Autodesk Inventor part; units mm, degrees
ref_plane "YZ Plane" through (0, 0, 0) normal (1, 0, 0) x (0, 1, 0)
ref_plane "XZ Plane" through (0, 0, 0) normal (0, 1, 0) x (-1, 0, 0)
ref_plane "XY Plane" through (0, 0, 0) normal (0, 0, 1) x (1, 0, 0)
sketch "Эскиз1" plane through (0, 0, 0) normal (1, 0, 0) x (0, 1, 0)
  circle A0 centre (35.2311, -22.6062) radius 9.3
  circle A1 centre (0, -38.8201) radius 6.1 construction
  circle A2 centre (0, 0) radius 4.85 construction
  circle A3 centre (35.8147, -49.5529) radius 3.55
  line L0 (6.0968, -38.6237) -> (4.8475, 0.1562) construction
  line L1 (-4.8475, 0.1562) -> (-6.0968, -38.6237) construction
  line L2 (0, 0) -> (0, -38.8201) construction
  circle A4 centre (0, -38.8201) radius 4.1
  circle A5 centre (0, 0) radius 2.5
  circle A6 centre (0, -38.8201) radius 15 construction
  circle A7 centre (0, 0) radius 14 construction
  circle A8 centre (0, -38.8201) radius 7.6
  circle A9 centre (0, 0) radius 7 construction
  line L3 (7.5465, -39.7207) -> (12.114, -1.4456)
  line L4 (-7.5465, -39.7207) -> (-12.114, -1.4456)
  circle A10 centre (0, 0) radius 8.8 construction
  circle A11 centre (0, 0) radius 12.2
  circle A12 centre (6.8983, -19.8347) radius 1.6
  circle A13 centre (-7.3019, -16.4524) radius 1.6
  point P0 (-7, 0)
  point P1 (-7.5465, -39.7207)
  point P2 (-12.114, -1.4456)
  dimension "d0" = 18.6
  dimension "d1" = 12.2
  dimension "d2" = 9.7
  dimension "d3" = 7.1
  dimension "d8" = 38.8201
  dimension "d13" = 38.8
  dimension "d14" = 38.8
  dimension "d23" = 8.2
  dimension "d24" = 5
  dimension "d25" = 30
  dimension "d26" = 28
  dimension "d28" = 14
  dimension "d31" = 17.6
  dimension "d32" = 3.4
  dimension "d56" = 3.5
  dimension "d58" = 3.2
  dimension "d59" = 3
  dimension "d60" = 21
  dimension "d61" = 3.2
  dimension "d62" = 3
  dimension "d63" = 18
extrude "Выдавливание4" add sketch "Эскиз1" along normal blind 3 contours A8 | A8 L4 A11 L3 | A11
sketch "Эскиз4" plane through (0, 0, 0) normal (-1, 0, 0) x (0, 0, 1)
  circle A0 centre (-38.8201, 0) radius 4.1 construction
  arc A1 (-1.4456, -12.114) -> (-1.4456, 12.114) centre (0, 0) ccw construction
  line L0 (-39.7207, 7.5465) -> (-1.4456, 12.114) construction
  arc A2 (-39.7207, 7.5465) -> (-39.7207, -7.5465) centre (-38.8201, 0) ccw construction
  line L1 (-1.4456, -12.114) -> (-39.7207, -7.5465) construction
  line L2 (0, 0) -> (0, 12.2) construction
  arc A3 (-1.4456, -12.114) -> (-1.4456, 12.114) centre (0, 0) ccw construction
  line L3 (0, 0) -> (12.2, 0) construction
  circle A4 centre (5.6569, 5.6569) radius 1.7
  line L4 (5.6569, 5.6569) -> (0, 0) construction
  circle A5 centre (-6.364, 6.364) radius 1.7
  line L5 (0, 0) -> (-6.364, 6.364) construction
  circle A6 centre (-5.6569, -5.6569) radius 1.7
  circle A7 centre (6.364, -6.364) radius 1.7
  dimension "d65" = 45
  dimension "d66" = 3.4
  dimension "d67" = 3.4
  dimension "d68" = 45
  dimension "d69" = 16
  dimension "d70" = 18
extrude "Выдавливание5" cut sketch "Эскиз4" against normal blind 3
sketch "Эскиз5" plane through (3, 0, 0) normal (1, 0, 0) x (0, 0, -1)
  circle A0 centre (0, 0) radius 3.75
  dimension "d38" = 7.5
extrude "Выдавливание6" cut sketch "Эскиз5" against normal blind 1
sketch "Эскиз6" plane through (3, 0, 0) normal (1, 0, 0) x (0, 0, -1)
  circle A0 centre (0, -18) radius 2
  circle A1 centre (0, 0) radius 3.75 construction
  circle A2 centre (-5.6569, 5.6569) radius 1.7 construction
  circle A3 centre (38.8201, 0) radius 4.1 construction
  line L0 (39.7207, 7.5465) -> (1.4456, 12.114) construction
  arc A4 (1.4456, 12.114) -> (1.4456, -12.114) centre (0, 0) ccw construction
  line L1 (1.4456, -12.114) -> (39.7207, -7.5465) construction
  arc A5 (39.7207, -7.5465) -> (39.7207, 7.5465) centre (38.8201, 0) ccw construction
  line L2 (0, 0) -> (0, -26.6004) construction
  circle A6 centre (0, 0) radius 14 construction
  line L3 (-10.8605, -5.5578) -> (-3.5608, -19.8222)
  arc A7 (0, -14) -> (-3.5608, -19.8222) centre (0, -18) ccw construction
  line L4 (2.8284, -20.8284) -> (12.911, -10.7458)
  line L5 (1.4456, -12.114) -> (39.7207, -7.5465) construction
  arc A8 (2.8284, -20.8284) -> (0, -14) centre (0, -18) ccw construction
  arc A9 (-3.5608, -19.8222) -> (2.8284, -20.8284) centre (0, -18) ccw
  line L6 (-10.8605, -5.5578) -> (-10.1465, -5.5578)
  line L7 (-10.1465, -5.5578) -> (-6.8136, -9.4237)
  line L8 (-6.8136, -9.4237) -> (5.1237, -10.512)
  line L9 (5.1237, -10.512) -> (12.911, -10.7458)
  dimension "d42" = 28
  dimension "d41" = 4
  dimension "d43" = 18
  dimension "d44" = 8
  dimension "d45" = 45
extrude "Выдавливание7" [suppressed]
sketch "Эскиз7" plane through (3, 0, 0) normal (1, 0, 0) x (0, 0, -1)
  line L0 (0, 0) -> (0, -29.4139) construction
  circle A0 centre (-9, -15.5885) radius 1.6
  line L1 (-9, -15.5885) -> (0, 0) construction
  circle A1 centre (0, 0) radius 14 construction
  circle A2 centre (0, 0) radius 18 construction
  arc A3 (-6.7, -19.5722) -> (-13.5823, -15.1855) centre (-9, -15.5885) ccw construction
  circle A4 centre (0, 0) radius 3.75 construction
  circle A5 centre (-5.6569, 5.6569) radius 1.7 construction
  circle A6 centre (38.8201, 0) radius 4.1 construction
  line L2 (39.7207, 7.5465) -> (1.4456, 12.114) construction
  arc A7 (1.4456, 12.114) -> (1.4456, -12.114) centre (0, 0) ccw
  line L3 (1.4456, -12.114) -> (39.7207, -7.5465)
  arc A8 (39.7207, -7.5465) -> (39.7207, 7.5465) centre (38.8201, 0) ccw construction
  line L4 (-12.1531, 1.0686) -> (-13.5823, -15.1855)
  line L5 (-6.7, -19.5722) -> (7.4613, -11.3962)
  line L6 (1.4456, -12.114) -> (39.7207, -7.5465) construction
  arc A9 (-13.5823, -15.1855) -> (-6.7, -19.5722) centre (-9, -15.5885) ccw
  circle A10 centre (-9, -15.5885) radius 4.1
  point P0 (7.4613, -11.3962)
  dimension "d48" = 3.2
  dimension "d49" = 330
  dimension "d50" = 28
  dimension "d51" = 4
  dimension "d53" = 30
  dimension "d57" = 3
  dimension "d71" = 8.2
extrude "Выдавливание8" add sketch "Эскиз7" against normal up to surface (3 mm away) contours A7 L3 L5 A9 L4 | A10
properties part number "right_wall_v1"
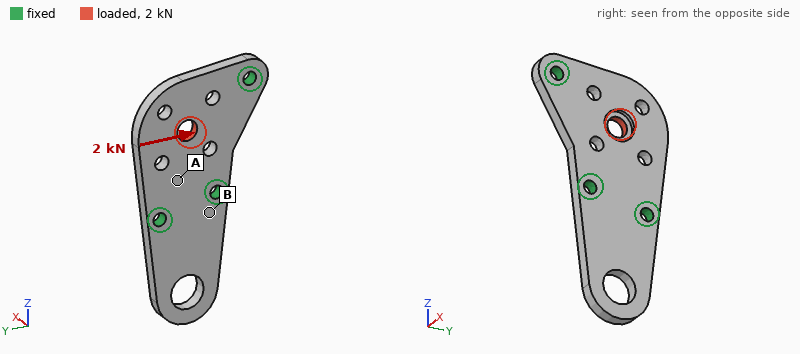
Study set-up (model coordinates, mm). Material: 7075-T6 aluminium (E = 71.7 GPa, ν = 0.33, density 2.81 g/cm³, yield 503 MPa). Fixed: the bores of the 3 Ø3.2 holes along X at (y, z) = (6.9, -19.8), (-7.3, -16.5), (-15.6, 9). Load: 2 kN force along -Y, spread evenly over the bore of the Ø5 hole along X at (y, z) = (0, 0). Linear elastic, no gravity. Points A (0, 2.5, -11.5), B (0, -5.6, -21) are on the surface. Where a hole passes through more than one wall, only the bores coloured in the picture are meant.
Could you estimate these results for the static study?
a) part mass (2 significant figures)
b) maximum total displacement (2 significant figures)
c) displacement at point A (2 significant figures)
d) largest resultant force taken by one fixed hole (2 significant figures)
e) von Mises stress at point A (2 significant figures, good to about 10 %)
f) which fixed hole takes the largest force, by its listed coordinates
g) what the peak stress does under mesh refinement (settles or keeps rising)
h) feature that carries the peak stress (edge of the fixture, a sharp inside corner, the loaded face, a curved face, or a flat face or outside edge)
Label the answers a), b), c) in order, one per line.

a) 9.2 g
b) 35 µm
c) 5.6 µm
d) 1.3 kN
e) 32 MPa
f) (-15.6, 9)
g) keeps rising
h) edge of the fixture
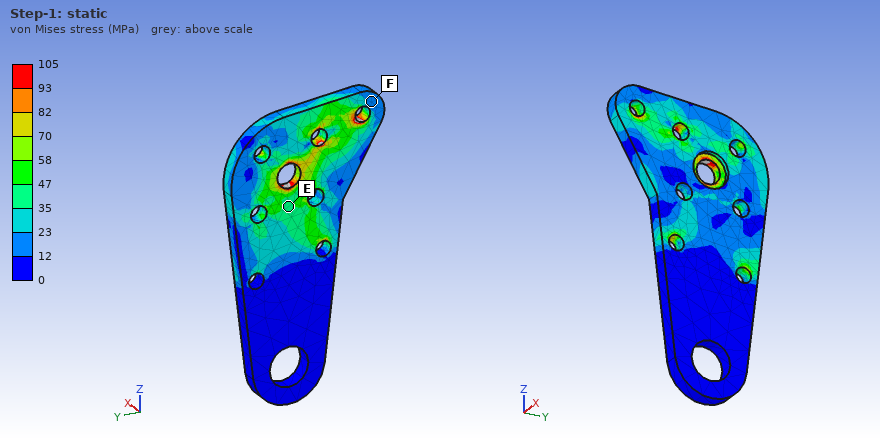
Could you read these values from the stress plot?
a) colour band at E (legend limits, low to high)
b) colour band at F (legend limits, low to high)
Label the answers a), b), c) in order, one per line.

a) 35 to 47 MPa
b) 12 to 23 MPa
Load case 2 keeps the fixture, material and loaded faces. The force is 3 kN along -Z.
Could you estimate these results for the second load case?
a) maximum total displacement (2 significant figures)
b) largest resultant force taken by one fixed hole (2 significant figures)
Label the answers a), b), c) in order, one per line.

a) 38 µm
b) 1.3 kN
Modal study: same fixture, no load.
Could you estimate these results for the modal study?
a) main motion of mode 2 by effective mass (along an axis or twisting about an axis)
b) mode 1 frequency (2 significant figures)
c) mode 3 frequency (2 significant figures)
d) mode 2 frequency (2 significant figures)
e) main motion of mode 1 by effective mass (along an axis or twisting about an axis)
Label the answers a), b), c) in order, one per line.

a) along X
b) 4500 Hz
c) 14 kHz
d) 6300 Hz
e) along X
